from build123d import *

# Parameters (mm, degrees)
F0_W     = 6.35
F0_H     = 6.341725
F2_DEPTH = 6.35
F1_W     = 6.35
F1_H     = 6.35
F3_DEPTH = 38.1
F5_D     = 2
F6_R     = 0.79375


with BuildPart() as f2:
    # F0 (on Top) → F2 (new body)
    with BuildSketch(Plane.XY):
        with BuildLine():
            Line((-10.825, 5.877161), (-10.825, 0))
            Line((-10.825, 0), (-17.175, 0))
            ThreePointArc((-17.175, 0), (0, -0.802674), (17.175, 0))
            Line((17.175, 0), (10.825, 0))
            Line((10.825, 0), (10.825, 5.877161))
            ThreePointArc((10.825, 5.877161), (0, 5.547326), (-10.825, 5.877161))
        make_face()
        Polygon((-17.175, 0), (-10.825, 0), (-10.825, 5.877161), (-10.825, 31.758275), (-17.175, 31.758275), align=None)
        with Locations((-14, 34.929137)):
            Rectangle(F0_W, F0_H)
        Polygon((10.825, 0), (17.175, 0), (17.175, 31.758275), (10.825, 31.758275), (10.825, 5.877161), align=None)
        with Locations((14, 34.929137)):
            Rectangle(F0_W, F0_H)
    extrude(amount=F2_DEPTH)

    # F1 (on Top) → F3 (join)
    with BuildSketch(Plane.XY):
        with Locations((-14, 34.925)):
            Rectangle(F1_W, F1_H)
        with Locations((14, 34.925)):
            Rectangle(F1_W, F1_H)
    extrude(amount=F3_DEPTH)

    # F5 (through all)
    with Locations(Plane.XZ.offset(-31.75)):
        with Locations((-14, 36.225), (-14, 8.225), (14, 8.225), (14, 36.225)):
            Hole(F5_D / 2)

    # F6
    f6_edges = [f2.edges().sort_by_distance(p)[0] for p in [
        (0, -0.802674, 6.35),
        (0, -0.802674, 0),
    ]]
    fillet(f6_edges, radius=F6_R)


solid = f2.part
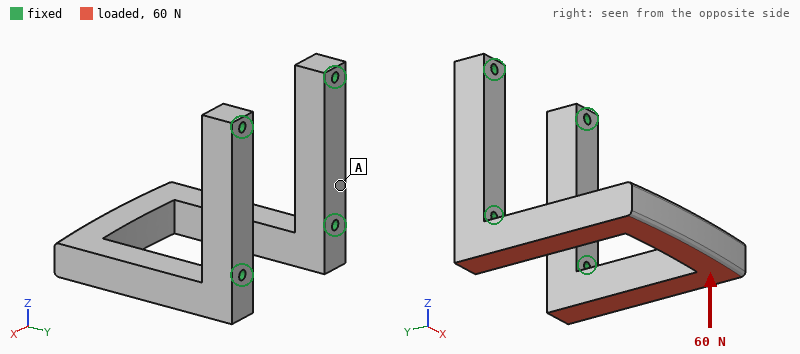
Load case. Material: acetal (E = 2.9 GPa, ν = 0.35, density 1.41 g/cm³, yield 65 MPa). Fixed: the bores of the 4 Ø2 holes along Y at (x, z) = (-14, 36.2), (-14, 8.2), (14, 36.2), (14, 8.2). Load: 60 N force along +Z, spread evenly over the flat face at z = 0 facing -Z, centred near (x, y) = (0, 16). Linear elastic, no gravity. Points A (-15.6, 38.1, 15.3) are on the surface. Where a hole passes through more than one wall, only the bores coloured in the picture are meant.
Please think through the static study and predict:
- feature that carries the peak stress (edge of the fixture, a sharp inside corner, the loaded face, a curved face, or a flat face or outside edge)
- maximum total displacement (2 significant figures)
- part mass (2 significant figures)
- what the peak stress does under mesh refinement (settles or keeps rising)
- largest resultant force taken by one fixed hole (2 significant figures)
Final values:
a sharp inside corner
0.68 mm
9.1 g
keeps rising
29 N
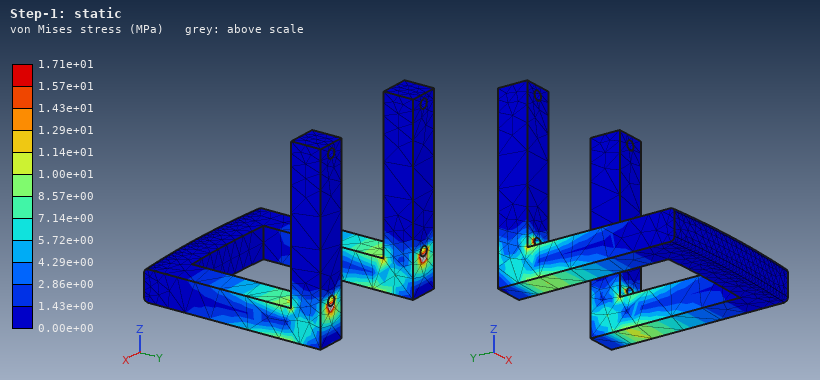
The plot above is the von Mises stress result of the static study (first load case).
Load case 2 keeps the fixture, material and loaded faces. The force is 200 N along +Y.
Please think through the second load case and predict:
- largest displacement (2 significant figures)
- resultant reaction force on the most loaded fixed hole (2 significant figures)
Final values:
0.62 mm
100 N
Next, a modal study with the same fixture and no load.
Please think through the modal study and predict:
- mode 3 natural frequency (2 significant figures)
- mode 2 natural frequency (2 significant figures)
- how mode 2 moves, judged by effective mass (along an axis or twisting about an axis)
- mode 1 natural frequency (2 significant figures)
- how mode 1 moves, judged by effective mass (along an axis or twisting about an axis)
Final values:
1600 Hz
1200 Hz
along X
720 Hz
along Z
